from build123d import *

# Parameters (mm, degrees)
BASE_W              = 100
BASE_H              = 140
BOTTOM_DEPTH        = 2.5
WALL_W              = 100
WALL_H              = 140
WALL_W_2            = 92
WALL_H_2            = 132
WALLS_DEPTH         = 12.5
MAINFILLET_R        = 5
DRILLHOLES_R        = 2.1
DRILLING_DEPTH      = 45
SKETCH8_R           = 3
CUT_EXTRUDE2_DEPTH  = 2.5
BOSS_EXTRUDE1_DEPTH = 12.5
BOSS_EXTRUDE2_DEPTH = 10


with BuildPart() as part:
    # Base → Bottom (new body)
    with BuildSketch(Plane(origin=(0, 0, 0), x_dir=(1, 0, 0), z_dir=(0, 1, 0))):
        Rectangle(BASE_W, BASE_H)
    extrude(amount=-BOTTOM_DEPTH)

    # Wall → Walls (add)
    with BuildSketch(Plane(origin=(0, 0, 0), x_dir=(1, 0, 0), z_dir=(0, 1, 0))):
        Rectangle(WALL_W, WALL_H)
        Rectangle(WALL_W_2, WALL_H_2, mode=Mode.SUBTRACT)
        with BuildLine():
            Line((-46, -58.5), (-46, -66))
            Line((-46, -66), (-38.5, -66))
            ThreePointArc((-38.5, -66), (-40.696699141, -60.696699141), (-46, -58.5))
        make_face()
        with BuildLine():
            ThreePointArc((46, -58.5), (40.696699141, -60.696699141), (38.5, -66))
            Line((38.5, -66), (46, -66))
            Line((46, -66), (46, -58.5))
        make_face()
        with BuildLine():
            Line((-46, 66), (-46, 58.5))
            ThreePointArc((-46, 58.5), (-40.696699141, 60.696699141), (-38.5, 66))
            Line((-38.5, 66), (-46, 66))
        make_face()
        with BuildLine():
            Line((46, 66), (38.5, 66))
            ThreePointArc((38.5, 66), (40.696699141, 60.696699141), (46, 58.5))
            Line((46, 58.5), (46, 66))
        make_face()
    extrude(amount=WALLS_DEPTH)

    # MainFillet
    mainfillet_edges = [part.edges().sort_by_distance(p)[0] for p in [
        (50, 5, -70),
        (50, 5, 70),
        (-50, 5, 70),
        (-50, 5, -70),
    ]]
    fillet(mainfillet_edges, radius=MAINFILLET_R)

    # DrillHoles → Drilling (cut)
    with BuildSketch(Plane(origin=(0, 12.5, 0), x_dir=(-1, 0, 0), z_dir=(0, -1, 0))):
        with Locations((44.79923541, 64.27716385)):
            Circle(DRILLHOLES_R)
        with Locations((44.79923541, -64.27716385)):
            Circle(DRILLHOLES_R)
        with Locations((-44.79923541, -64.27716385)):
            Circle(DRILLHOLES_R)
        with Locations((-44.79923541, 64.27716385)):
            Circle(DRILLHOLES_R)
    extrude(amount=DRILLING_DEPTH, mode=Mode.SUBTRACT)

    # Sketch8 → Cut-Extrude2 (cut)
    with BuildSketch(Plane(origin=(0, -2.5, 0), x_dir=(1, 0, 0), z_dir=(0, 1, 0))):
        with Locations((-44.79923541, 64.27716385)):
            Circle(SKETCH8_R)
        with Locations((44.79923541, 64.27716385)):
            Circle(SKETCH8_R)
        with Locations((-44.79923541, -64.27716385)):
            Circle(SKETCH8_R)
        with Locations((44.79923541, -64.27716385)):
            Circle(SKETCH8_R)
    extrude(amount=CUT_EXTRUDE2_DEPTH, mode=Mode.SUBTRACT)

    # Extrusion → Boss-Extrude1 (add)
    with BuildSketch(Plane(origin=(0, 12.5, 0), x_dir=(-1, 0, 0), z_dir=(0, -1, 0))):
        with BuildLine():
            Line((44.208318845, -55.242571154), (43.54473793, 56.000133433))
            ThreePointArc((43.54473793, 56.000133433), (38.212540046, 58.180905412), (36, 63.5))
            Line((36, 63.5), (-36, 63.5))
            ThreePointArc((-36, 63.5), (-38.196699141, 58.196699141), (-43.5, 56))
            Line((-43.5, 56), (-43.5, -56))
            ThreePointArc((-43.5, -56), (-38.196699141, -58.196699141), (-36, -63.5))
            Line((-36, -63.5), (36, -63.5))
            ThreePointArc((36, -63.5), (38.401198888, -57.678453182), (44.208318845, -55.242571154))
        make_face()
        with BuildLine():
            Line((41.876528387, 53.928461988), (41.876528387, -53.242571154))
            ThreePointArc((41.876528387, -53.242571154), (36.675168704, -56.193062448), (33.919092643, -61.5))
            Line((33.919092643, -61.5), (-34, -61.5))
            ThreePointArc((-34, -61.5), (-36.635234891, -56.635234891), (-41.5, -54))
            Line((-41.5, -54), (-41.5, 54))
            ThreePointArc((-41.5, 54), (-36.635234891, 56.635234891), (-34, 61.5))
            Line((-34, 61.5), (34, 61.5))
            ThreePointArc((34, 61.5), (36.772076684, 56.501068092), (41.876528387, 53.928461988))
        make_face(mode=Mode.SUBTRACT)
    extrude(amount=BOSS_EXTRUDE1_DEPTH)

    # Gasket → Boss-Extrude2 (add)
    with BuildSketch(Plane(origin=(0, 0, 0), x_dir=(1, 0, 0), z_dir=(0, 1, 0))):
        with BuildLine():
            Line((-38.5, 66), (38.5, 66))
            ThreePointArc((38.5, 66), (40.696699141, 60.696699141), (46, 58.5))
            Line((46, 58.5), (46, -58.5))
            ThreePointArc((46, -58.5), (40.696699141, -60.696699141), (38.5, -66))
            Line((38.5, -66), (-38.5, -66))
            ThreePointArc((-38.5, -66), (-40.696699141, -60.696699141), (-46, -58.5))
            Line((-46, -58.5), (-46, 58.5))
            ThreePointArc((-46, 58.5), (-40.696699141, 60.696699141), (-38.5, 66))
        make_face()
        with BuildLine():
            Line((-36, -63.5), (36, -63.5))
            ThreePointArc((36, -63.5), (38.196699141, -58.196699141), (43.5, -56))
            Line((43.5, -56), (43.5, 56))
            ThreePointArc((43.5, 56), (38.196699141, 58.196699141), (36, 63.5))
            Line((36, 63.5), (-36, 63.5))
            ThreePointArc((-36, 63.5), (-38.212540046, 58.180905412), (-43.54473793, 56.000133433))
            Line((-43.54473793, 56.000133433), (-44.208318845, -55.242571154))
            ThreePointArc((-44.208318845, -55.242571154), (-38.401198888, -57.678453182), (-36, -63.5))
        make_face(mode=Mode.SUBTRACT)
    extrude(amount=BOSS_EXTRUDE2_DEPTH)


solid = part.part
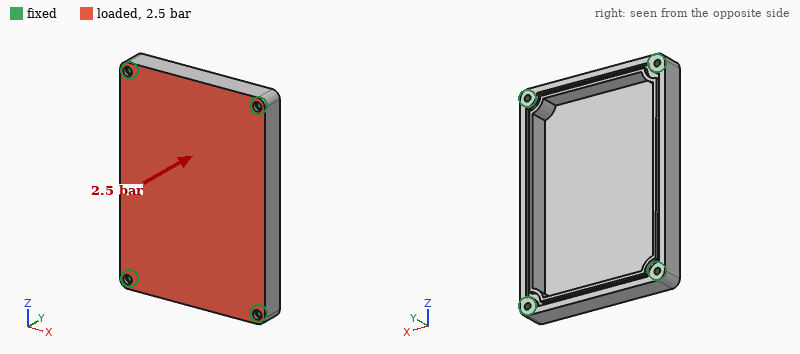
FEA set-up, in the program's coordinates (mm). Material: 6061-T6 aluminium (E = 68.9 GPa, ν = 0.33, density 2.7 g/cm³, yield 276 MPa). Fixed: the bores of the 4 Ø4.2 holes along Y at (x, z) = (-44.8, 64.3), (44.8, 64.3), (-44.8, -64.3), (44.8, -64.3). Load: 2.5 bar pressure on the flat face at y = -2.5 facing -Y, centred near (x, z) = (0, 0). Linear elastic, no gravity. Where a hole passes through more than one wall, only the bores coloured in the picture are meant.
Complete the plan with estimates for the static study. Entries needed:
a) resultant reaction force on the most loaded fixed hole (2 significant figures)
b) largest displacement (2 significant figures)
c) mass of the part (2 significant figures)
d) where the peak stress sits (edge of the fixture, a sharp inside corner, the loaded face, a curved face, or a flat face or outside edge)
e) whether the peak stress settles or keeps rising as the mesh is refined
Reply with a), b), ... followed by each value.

a) 1.1 kN
b) 0.41 mm
c) 220 g
d) edge of the fixture
e) keeps rising
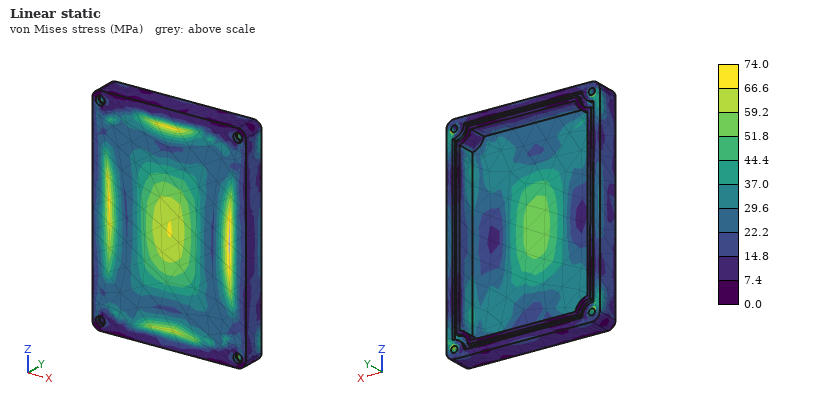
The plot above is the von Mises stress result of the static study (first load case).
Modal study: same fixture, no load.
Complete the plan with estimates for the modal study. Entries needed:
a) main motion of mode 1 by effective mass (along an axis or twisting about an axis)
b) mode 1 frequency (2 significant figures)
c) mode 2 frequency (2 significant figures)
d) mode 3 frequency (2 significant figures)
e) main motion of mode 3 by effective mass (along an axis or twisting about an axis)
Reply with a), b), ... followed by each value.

a) along Y
b) 1900 Hz
c) 3300 Hz
d) 3600 Hz
e) twisting about Z
